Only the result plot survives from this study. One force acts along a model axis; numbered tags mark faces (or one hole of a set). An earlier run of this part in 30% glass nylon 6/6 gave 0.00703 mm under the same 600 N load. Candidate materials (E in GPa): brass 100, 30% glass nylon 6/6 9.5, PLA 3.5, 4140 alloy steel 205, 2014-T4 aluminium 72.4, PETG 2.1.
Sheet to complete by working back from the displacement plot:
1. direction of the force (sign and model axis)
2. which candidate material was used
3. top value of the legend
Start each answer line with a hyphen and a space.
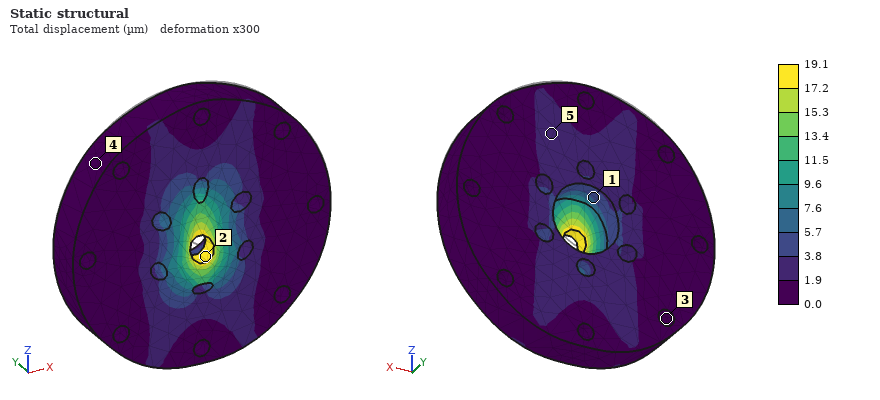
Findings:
- -Z
- PLA
- 19.1 µm
